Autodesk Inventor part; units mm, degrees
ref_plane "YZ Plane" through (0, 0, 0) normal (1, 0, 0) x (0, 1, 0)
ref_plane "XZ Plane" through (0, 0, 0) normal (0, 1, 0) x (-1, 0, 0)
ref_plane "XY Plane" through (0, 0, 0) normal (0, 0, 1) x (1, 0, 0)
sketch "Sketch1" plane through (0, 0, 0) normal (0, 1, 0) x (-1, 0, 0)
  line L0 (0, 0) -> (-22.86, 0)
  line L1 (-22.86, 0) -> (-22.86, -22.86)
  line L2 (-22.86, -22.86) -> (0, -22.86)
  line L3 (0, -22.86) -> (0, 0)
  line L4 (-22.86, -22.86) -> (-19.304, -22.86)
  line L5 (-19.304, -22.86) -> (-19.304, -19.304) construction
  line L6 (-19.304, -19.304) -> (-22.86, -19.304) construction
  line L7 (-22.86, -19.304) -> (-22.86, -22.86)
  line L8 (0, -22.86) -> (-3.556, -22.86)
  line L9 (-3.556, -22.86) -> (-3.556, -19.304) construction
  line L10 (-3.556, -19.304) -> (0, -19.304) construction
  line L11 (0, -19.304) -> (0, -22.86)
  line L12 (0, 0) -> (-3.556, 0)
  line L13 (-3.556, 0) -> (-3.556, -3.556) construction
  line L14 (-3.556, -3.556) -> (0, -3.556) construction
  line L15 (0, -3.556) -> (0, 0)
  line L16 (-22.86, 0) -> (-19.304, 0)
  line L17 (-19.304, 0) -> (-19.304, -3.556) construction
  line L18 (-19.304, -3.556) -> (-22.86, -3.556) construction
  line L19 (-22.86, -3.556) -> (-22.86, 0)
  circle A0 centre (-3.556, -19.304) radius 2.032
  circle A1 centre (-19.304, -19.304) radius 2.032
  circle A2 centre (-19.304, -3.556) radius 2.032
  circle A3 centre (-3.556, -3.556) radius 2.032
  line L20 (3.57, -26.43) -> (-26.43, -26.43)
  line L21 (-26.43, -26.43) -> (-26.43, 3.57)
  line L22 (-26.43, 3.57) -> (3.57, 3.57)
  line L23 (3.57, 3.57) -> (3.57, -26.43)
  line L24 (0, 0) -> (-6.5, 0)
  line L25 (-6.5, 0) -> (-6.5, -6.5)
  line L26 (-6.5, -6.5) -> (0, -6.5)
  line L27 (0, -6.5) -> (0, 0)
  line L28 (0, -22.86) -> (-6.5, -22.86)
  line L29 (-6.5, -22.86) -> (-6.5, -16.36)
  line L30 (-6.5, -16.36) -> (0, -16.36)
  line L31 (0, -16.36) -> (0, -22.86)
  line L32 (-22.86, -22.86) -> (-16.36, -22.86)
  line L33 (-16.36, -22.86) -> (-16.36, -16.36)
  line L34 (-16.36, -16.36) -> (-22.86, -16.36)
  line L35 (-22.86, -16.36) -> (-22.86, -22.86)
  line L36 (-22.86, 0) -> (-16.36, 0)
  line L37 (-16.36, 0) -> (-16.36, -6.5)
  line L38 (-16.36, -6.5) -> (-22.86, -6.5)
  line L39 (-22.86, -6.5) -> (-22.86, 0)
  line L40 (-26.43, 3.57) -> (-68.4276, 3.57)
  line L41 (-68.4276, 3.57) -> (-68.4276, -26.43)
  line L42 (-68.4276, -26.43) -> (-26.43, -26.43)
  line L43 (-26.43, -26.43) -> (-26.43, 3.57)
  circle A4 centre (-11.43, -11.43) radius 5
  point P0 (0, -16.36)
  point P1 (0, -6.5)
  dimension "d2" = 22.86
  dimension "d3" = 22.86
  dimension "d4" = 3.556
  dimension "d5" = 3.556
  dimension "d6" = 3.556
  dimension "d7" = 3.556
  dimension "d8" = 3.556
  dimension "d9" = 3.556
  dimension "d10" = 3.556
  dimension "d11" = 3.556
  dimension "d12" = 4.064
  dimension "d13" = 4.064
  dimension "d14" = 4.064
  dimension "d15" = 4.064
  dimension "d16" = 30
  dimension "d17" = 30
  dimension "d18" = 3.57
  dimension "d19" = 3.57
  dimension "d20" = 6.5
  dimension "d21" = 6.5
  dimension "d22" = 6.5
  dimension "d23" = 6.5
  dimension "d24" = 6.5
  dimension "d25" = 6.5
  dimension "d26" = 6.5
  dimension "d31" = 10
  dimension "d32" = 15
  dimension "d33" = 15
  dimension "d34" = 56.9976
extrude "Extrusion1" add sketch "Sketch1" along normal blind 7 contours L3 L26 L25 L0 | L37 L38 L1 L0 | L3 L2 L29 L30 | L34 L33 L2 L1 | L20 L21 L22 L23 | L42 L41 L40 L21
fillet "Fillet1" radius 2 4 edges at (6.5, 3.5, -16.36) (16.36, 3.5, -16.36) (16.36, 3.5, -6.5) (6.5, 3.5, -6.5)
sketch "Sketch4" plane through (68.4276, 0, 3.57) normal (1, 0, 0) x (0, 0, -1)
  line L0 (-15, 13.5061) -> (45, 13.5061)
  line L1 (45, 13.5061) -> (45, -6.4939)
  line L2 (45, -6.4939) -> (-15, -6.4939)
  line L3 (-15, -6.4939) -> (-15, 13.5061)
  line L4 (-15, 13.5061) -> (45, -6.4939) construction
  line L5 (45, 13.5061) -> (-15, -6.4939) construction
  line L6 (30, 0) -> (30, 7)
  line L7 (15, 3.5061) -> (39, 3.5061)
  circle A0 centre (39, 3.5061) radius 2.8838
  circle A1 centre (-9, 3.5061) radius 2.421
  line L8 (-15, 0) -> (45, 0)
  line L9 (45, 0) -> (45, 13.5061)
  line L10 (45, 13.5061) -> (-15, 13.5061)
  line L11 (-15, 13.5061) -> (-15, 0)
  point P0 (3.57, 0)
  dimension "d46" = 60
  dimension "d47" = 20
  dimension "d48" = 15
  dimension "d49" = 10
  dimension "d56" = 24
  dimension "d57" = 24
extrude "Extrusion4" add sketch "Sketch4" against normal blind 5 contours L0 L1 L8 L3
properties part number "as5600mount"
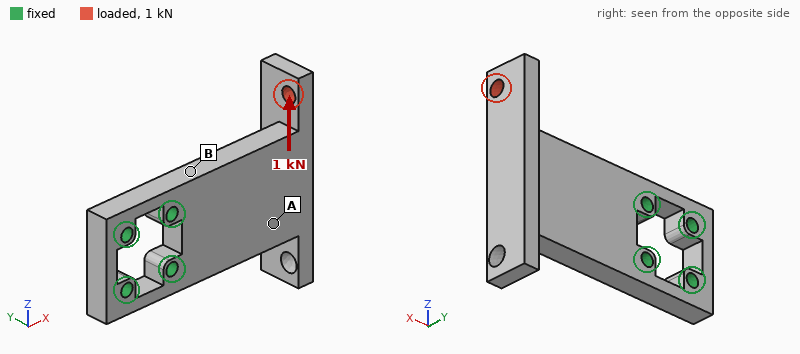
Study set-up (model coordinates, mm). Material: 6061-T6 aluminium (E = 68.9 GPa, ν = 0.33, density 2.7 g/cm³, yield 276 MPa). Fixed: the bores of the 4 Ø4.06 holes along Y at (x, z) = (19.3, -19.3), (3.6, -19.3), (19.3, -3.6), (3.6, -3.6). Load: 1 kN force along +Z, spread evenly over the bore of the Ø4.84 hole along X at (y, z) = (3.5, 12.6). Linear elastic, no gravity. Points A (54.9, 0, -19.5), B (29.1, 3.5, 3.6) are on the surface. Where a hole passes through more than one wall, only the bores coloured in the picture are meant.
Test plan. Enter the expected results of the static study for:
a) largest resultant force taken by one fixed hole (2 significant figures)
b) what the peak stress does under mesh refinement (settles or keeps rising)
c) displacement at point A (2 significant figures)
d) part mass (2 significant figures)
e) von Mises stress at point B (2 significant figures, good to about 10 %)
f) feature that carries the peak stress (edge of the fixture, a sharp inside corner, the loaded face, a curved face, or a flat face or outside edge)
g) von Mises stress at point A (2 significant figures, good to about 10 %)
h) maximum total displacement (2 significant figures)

2.0 kN
keeps rising
34 µm
41 g
29 MPa
edge of the fixture
10 MPa
77 µm
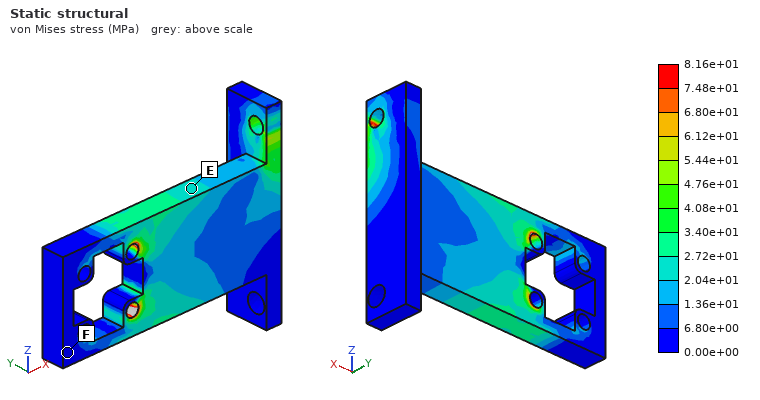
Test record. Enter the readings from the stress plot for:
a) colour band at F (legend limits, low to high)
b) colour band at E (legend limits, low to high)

0.00e+00 to 6.80e+00 MPa
2.04e+01 to 2.72e+01 MPa
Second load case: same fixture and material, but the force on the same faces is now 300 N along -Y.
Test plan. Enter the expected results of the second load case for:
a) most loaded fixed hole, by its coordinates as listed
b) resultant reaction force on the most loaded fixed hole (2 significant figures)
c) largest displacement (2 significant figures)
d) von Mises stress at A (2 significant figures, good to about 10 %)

(19.3, -3.6)
520 N
0.34 mm
25 MPa
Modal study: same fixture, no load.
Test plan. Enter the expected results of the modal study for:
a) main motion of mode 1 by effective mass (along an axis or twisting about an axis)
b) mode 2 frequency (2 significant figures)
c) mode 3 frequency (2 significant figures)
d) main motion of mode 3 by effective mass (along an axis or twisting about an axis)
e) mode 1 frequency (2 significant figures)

along Y
3600 Hz
5300 Hz
along Z
1600 Hz
